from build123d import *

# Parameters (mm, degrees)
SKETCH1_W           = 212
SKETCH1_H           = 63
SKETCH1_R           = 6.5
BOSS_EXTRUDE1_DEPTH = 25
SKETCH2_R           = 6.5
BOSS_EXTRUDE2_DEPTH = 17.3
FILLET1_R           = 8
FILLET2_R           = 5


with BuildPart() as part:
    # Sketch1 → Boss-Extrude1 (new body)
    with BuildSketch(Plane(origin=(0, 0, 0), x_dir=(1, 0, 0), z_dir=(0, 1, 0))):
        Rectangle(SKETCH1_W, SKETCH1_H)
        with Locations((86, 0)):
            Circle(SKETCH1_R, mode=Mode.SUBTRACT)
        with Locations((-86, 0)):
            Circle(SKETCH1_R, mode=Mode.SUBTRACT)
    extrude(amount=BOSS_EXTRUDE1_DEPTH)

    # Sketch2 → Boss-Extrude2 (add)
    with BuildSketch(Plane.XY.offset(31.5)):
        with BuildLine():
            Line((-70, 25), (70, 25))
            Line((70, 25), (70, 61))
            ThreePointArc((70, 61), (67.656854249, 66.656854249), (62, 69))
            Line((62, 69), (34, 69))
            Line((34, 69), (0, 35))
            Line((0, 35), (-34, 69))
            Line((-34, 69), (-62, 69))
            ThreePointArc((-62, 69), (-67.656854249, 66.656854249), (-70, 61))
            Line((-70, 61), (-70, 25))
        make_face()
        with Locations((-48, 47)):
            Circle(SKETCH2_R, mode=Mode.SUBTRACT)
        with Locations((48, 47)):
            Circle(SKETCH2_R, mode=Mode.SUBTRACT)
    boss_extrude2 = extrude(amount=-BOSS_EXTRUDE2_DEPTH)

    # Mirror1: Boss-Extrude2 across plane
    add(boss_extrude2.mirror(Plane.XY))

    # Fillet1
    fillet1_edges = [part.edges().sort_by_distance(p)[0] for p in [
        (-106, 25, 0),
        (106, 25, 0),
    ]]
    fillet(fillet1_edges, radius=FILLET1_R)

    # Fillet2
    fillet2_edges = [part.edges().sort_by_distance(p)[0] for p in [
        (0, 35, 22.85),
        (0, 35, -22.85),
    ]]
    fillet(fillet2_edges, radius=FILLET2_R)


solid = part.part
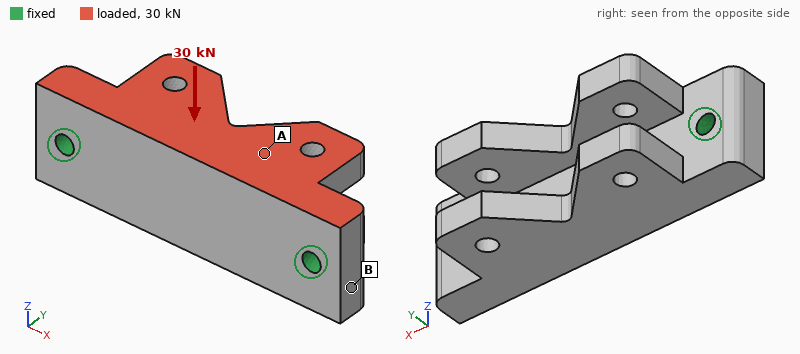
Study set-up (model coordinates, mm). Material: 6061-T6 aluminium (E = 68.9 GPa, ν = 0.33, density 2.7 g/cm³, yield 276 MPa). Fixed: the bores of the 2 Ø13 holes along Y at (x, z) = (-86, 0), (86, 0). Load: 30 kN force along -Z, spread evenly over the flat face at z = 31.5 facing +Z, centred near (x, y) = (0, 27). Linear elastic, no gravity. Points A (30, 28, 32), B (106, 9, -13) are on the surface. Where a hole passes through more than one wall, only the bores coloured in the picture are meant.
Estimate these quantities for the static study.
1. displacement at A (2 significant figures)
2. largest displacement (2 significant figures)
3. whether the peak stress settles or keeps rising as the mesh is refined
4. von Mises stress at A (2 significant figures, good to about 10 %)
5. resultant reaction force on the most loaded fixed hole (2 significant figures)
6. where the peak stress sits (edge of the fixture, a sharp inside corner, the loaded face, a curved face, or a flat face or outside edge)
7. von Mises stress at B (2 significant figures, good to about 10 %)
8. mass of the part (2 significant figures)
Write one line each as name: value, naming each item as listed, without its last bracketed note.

displacement at A: 0.087 mm
largest displacement: 0.20 mm
whether the peak stress settles or keeps rising as the mesh is refined: keeps rising
von Mises stress at A: 31 MPa
resultant reaction force on the most loaded fixed hole: 15 kN
where the peak stress sits: edge of the fixture
von Mises stress at B: 8.7 MPa
mass of the part: 1.3 kg
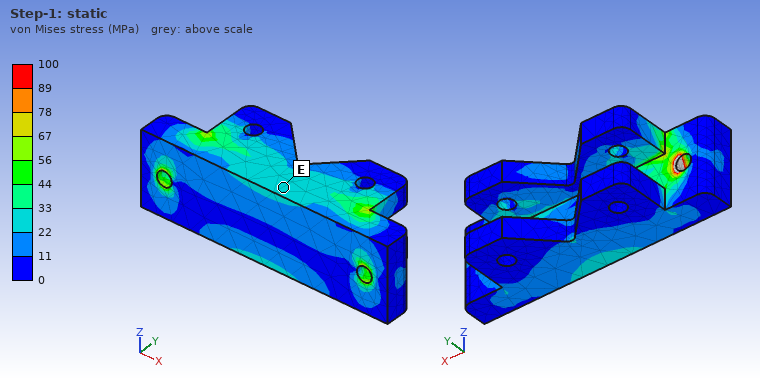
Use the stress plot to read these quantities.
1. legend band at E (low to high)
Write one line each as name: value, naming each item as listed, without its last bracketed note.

legend band at E: 22 to 33 MPa
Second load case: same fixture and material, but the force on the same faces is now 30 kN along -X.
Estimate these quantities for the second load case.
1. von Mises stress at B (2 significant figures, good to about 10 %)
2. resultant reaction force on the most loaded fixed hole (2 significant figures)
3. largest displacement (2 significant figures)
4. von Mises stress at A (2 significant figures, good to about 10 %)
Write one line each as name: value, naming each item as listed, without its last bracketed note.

von Mises stress at B: 5.9 MPa
resultant reaction force on the most loaded fixed hole: 16 kN
largest displacement: 31 µm
von Mises stress at A: 9.5 MPa
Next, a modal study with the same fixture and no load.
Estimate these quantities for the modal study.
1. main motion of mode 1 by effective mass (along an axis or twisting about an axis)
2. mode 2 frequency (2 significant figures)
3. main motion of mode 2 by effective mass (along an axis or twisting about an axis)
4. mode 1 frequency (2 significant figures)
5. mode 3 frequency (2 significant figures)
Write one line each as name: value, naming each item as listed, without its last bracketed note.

main motion of mode 1 by effective mass: along Z
mode 2 frequency: 3600 Hz
main motion of mode 2 by effective mass: along Y
mode 1 frequency: 2700 Hz
mode 3 frequency: 4600 Hz
